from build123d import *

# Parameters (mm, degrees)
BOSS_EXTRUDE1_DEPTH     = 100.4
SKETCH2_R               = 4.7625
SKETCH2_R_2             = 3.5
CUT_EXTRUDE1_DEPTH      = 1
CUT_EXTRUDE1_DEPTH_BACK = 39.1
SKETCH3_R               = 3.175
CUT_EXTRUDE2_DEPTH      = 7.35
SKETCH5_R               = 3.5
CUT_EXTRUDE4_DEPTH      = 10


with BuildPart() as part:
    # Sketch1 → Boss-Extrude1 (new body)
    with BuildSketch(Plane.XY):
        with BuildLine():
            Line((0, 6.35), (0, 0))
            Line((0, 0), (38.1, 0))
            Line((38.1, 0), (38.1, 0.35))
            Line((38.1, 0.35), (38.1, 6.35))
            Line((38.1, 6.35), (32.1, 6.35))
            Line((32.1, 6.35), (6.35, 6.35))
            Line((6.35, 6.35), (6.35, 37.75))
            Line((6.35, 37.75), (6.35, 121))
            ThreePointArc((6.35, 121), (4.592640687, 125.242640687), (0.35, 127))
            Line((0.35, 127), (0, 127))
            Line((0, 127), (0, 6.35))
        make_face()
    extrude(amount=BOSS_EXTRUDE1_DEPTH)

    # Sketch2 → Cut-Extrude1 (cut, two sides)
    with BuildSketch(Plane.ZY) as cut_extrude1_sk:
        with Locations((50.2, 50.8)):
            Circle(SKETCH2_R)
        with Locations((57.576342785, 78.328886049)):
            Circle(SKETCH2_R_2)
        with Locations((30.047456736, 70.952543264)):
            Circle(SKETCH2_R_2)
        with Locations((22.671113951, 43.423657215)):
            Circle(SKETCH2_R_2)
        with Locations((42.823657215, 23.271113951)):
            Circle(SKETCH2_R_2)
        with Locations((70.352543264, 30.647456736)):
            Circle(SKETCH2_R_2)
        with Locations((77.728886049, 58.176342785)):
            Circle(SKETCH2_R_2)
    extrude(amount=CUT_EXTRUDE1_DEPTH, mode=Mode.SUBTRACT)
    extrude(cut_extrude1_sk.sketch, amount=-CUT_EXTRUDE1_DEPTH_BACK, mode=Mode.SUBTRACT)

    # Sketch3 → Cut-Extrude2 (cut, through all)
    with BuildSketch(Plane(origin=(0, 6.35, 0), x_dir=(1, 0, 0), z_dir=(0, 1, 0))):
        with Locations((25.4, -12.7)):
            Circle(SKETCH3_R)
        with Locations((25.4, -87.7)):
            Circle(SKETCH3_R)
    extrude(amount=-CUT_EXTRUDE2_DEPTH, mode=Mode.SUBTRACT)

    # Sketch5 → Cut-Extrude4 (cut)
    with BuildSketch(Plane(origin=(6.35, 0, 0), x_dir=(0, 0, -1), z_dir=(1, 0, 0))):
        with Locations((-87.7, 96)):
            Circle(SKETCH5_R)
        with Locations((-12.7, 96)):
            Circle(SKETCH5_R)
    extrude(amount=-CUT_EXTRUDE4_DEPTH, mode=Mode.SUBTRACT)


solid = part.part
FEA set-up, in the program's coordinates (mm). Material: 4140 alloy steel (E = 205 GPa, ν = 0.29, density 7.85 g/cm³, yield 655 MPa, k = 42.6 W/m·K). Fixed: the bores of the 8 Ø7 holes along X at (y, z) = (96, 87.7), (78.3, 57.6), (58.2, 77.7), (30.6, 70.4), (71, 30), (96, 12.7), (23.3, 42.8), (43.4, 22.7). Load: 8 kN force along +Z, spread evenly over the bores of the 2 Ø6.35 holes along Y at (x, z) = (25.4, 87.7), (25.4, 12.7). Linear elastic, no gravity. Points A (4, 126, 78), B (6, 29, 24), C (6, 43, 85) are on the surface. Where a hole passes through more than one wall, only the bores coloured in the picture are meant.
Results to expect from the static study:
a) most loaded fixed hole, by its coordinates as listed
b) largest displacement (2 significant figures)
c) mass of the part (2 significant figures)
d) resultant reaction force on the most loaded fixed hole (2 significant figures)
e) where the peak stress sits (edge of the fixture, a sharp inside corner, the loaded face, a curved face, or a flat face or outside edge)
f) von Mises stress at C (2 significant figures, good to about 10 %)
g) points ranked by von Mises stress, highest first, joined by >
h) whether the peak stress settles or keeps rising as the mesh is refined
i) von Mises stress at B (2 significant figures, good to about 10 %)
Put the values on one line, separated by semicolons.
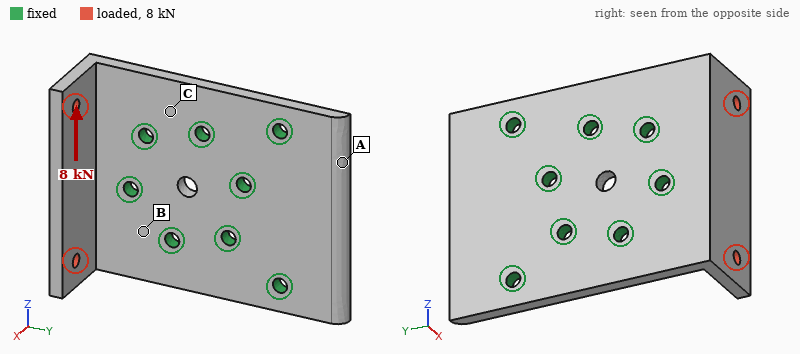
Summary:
(23.3, 42.8); 0.20 mm; 770 g; 5.8 kN; edge of the fixture; 55 MPa; B > C > A; keeps rising; 97 MPa
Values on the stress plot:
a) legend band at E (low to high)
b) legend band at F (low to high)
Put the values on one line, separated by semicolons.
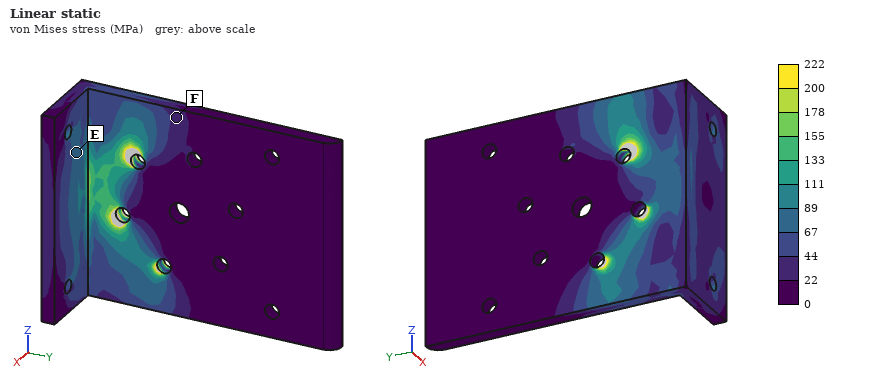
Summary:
67 to 89 MPa; 22 to 44 MPa
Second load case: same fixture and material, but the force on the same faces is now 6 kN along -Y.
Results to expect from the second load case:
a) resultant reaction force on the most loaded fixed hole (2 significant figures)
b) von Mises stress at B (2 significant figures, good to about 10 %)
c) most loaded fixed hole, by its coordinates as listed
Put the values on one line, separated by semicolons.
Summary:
3.2 kN; 80 MPa; (23.3, 42.8)
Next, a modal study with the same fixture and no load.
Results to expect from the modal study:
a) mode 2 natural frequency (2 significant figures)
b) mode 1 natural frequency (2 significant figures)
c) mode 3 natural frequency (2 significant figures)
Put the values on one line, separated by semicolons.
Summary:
2400 Hz; 2100 Hz; 4300 Hz
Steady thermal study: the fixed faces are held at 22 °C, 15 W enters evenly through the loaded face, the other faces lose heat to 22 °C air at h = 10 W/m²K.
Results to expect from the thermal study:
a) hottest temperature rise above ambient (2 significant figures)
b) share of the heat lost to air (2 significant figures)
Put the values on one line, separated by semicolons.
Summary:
33 K; 15 %
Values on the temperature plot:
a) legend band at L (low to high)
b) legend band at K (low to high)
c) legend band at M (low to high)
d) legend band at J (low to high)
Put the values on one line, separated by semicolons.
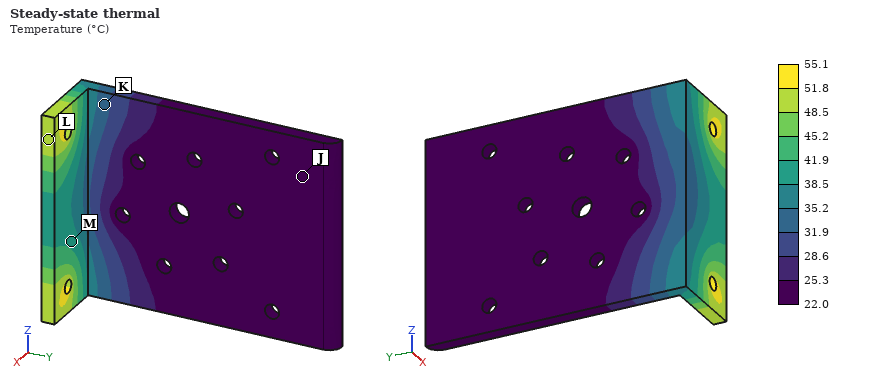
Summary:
48.5 to 51.8 °C; 31.9 to 35.2 °C; 38.5 to 41.9 °C; 22.0 to 25.3 °C
